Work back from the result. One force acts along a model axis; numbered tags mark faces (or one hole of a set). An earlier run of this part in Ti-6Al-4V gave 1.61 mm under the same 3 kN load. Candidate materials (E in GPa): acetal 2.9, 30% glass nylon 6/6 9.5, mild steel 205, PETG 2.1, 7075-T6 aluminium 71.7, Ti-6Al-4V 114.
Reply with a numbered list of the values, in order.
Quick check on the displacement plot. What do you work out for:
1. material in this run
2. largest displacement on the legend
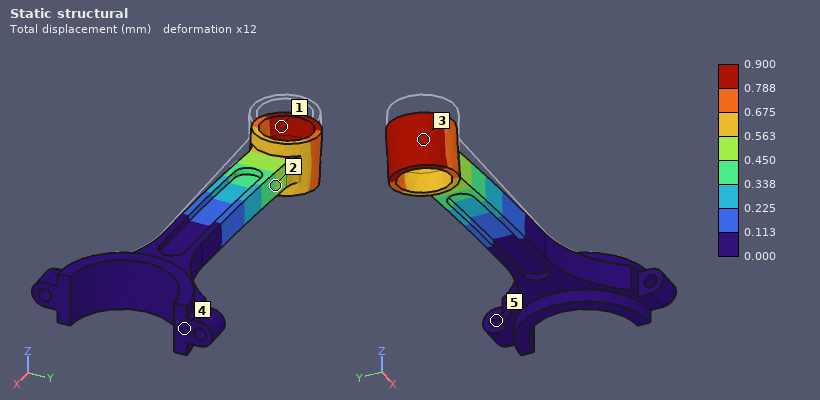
1. mild steel
2. 0.900 mm
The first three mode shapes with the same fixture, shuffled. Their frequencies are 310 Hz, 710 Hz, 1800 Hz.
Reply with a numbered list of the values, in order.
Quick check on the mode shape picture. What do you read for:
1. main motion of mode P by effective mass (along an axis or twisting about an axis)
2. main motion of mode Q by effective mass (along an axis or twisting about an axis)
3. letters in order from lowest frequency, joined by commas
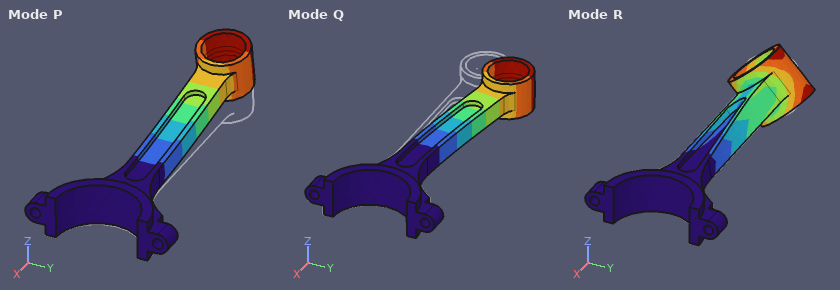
1. along Z
2. along Y
3. P, Q, R
